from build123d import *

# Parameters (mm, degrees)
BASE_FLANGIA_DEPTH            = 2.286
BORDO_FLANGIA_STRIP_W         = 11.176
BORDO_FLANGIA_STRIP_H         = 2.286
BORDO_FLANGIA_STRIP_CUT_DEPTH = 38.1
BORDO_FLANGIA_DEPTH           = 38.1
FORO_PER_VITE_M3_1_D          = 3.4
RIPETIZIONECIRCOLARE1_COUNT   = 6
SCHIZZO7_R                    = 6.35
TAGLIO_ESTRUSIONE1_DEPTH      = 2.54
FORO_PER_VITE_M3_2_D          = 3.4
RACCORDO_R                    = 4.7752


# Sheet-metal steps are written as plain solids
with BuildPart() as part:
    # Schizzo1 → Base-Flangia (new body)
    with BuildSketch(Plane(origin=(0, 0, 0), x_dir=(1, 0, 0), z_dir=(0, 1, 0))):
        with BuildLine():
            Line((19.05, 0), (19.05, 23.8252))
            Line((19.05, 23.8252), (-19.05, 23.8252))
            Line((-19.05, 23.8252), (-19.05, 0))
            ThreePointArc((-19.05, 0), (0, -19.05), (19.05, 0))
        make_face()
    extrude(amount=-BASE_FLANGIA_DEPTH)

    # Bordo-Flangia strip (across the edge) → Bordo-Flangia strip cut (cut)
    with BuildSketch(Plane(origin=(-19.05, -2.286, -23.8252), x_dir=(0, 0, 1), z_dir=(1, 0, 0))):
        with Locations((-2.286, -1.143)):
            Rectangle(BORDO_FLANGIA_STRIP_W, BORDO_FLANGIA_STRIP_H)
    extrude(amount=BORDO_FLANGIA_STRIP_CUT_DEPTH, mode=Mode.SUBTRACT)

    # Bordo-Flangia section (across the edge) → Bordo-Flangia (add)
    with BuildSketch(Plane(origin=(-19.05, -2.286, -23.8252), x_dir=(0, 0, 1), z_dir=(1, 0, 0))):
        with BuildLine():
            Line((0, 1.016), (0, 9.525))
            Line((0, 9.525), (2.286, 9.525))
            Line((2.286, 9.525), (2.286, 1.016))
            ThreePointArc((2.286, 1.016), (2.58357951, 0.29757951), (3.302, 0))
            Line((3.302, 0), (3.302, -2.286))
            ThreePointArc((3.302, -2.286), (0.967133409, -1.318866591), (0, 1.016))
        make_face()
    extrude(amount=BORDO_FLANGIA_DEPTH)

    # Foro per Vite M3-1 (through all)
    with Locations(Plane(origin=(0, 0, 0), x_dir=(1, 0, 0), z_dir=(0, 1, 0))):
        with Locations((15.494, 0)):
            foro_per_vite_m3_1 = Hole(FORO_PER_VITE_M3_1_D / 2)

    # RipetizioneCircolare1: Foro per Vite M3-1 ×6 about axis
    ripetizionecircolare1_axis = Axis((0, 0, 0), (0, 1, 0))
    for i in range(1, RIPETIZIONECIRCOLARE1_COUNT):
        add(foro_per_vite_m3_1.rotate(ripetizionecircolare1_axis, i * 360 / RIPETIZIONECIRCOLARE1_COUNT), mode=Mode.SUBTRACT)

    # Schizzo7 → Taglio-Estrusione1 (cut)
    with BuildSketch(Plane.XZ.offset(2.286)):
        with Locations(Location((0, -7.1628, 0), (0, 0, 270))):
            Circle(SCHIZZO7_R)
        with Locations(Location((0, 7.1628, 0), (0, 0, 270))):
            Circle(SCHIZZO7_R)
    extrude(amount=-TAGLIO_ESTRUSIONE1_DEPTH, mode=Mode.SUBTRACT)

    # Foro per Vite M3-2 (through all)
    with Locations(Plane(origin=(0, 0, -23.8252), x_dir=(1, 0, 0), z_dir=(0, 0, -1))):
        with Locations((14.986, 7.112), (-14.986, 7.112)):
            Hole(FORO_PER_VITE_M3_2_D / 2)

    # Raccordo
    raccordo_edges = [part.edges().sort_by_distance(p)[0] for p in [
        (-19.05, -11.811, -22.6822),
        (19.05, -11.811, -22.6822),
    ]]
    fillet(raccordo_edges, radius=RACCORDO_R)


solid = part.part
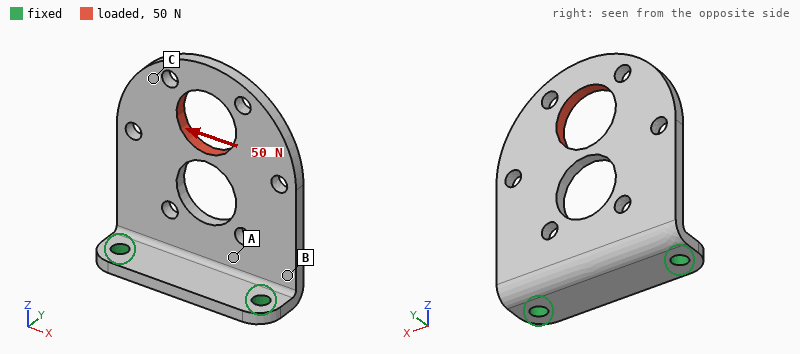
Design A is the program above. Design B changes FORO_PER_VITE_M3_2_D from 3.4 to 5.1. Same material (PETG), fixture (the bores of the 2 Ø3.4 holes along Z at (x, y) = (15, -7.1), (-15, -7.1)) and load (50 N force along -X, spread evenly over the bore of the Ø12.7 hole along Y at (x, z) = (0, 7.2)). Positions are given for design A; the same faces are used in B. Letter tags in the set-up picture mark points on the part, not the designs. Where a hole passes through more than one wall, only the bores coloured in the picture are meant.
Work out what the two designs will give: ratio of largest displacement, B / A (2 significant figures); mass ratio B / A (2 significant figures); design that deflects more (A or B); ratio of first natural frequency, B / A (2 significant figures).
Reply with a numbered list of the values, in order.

1. 0.74
2. 0.98
3. A
4. 1.0
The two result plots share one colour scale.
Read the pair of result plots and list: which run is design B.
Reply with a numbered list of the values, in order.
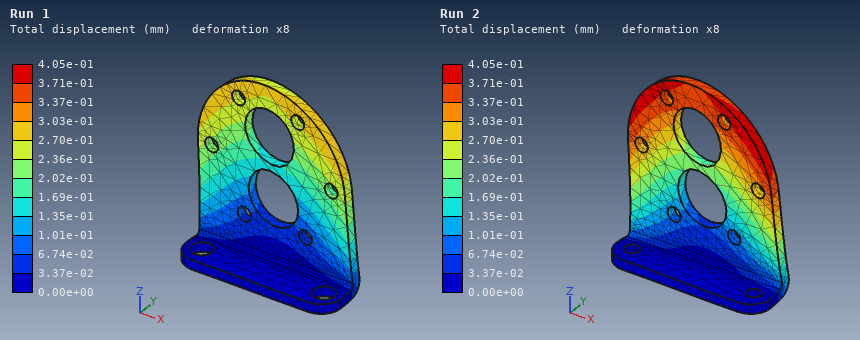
1. Run 1
